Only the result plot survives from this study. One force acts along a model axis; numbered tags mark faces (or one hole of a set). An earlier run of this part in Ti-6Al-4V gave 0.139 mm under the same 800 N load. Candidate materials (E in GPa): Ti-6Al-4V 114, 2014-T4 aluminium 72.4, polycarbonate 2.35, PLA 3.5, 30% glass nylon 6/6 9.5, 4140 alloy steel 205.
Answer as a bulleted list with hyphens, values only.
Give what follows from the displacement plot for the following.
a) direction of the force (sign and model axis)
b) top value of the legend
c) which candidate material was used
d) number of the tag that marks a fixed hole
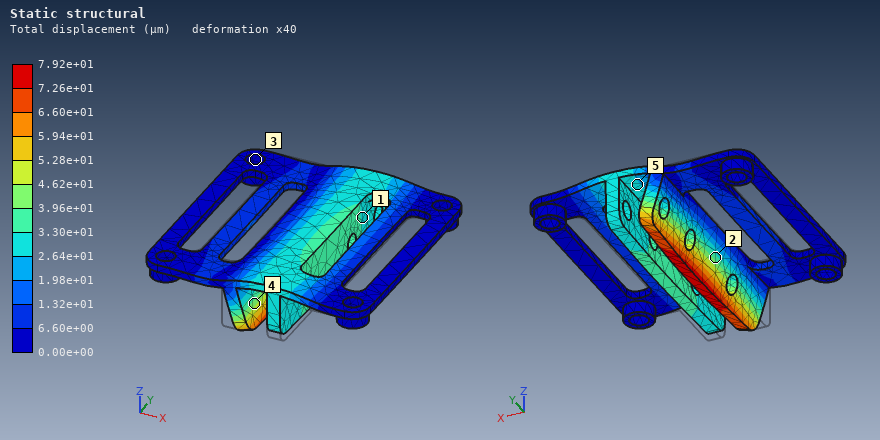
- +X
- 7.92e+01 µm
- 4140 alloy steel
- 3
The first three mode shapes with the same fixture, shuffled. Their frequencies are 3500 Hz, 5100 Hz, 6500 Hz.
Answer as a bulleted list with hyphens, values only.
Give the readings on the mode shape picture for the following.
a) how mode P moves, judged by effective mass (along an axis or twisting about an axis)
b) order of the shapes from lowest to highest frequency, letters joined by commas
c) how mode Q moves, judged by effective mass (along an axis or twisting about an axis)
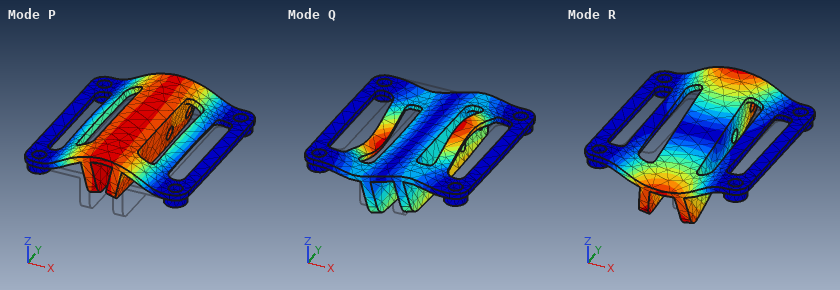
- along Z
- P, R, Q
- along X
